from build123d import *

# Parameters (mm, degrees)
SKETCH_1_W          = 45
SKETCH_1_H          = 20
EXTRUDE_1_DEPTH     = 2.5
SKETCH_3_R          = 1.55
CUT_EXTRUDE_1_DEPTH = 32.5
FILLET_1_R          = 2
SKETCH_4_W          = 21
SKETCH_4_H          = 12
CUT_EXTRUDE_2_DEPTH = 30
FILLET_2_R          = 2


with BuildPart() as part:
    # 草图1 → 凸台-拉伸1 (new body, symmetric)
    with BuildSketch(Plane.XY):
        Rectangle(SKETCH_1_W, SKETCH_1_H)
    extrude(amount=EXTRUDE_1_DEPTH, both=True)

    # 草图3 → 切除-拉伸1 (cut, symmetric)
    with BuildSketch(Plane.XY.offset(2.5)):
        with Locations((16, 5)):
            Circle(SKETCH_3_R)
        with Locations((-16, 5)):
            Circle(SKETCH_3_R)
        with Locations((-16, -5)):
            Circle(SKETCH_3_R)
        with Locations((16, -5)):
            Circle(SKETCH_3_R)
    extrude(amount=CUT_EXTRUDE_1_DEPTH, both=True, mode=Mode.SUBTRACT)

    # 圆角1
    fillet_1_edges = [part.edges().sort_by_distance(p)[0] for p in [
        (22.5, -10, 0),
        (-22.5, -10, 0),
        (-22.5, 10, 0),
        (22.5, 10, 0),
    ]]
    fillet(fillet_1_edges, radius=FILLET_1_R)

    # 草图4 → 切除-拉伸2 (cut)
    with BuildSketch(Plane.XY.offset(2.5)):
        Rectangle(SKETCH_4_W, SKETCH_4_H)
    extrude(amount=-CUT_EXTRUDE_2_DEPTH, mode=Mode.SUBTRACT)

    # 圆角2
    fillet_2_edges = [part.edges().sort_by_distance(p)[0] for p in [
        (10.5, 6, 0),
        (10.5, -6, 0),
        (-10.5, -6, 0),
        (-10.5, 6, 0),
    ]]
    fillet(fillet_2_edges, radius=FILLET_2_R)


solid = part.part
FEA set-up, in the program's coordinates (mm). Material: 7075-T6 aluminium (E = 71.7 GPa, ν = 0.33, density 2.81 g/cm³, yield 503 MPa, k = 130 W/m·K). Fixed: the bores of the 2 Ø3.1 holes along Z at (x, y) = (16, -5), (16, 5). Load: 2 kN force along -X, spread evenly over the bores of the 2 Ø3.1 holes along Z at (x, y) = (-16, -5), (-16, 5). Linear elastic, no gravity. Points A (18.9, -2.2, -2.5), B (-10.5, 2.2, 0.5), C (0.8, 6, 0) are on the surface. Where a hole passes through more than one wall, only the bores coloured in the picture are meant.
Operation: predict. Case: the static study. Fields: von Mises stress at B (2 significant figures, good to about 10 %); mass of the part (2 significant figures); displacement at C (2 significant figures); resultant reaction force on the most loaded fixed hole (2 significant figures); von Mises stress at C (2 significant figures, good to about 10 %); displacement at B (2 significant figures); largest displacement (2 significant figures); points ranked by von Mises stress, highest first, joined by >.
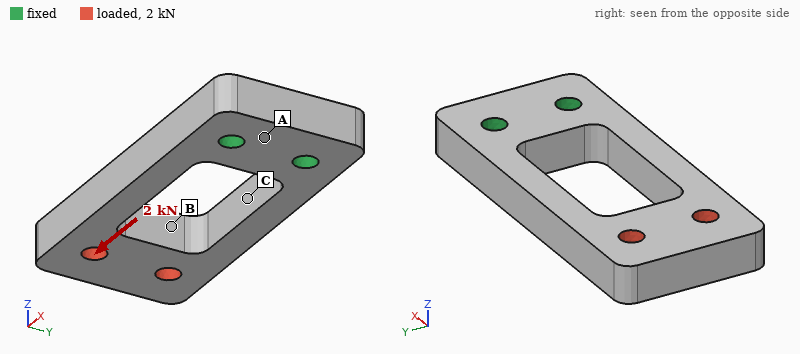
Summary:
45 MPa
8.7 g
14 µm
1.0 kN
65 MPa
25 µm
26 µm
C > B > A
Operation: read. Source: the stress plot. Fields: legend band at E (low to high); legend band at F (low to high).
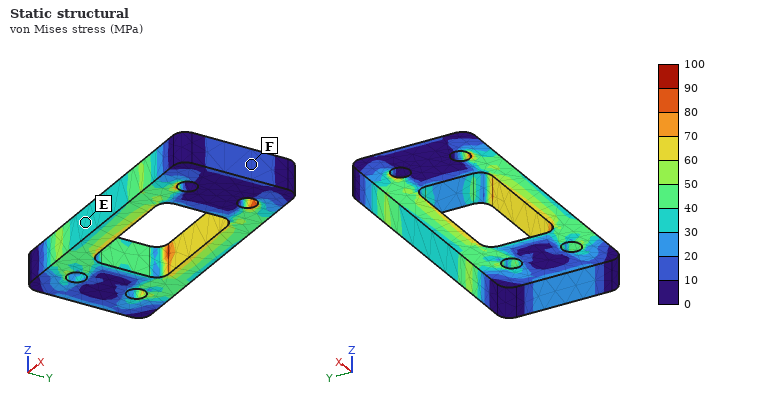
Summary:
30 to 40 MPa
10 to 20 MPa
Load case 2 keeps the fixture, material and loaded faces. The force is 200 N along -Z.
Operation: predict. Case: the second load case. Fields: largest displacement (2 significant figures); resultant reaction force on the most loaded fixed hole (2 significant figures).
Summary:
0.40 mm
100 N
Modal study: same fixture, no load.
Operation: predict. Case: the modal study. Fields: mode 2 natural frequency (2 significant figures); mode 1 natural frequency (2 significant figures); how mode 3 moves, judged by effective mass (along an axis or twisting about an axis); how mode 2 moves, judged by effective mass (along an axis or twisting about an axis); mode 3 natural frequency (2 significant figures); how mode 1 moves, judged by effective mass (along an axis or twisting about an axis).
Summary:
4100 Hz
2100 Hz
twisting about X
along Y
6600 Hz
along Z
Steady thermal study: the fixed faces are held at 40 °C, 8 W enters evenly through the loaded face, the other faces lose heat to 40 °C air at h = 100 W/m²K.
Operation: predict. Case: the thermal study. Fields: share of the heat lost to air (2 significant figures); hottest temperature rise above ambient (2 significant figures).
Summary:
38 %
30 K
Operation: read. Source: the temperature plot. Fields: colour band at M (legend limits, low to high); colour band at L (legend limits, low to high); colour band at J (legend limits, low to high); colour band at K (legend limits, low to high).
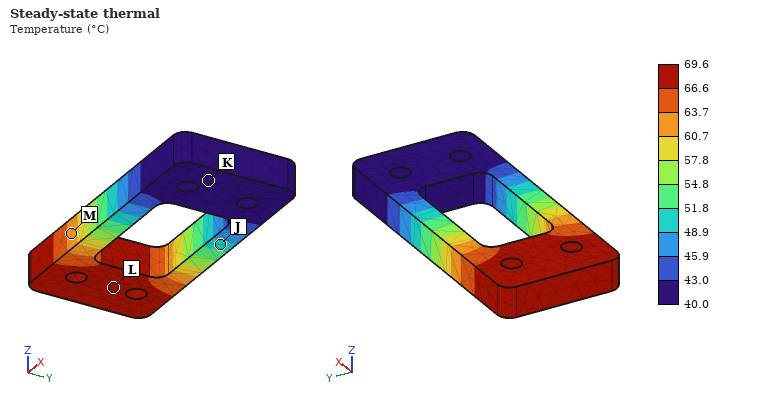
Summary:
60.7 to 63.7 °C
66.6 to 69.6 °C
48.9 to 51.8 °C
40.0 to 43.0 °C
